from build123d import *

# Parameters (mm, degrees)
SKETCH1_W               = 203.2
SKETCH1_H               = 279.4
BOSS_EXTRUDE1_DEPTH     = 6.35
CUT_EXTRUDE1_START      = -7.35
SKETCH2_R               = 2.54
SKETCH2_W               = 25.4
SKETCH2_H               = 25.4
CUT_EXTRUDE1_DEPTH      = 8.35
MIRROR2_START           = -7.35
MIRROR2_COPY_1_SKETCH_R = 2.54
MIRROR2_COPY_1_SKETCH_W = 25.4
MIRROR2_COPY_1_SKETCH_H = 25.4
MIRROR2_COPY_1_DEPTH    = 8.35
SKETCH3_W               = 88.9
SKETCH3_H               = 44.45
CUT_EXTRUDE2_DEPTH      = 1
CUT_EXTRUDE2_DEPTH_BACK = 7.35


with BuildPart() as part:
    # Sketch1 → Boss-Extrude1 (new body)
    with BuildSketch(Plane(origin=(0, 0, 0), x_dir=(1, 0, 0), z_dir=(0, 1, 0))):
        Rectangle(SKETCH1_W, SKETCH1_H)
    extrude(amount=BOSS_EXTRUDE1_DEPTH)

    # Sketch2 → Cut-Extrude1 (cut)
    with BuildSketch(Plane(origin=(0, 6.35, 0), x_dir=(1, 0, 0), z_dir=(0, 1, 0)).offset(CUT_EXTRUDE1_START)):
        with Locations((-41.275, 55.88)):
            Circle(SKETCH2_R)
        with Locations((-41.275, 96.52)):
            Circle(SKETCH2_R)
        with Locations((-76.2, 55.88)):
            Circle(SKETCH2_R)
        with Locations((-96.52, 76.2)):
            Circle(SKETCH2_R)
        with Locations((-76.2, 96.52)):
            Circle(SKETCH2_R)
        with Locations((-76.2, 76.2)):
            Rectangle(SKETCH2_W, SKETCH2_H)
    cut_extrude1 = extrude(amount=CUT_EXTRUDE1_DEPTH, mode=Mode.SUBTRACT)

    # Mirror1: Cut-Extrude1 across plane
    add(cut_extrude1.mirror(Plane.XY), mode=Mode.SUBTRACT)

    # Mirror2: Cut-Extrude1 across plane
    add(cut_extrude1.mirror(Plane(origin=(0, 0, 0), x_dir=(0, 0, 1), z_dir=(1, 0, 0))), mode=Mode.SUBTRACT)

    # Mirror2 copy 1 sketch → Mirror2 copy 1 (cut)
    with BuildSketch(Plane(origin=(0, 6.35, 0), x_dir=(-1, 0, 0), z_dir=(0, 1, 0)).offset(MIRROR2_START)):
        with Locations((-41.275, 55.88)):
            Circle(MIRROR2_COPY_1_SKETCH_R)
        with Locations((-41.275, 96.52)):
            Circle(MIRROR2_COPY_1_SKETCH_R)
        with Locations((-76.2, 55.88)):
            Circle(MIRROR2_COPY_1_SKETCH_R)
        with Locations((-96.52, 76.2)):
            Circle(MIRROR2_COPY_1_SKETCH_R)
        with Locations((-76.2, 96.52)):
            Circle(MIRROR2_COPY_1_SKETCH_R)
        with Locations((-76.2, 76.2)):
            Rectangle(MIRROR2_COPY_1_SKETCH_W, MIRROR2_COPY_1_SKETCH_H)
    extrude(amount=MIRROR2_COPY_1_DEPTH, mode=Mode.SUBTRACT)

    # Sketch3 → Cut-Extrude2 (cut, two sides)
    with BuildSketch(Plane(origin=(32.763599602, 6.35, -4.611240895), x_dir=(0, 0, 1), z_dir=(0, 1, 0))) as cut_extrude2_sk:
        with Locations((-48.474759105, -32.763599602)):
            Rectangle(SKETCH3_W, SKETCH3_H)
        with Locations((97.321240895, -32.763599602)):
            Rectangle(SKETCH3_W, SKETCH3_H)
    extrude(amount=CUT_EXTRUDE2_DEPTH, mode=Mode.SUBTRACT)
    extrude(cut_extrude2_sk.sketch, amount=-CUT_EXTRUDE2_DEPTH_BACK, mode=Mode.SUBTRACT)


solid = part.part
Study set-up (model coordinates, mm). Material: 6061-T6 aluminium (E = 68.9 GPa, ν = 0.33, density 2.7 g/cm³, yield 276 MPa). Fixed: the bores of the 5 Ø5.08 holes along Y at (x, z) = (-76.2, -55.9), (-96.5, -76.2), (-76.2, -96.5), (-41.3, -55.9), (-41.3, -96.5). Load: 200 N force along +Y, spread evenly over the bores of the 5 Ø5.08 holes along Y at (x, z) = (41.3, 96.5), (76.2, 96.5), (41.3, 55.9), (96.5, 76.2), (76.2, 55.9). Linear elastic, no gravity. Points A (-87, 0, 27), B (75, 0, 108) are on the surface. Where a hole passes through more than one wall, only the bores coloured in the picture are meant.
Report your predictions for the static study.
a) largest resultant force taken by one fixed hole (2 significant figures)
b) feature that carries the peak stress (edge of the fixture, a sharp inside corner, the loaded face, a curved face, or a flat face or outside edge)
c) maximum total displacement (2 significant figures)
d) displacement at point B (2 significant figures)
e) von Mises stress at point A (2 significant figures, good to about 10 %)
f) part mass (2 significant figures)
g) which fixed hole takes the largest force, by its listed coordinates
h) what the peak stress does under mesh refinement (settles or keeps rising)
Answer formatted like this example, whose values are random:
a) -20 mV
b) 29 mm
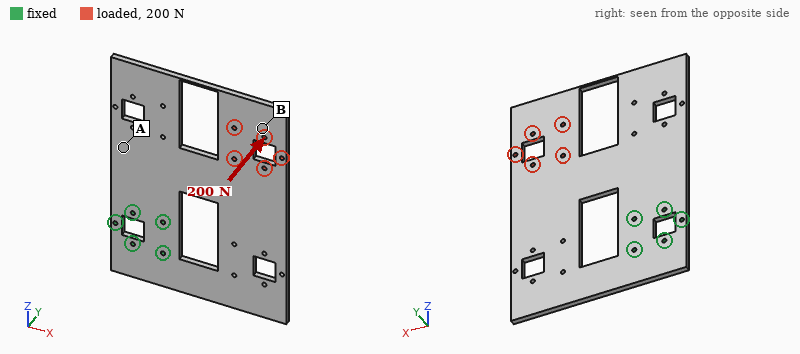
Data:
a) 680 N
b) edge of the fixture
c) 3.7 mm
d) 2.9 mm
e) 19 MPa
f) 790 g
g) (-41.3, -55.9)
h) keeps rising
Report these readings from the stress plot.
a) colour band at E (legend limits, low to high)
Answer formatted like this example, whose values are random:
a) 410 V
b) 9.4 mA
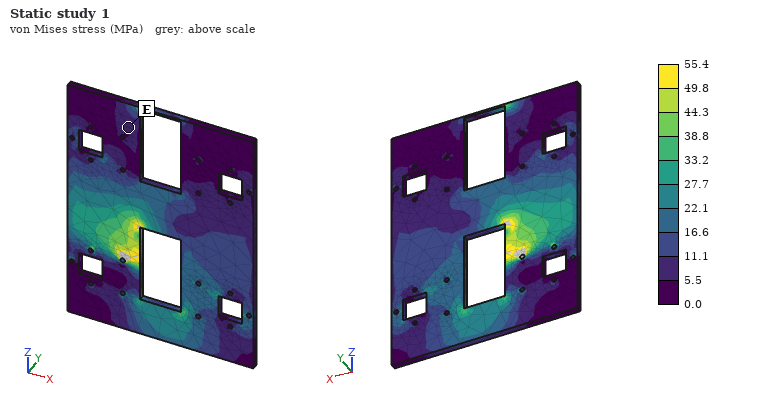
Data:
a) 5.5 to 11.1 MPa
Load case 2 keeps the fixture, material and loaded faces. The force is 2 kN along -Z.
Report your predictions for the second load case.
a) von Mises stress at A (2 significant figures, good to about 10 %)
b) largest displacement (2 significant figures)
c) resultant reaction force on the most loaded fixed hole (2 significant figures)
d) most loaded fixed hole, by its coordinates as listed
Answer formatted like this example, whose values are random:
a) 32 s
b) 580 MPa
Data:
a) 3.3 MPa
b) 0.14 mm
c) 3.1 kN
d) (-41.3, -55.9)
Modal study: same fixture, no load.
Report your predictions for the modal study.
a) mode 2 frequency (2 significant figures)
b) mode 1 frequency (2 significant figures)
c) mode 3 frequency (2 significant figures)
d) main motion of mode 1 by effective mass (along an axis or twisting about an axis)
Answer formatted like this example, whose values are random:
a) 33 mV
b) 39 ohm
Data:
a) 170 Hz
b) 97 Hz
c) 310 Hz
d) along Y
